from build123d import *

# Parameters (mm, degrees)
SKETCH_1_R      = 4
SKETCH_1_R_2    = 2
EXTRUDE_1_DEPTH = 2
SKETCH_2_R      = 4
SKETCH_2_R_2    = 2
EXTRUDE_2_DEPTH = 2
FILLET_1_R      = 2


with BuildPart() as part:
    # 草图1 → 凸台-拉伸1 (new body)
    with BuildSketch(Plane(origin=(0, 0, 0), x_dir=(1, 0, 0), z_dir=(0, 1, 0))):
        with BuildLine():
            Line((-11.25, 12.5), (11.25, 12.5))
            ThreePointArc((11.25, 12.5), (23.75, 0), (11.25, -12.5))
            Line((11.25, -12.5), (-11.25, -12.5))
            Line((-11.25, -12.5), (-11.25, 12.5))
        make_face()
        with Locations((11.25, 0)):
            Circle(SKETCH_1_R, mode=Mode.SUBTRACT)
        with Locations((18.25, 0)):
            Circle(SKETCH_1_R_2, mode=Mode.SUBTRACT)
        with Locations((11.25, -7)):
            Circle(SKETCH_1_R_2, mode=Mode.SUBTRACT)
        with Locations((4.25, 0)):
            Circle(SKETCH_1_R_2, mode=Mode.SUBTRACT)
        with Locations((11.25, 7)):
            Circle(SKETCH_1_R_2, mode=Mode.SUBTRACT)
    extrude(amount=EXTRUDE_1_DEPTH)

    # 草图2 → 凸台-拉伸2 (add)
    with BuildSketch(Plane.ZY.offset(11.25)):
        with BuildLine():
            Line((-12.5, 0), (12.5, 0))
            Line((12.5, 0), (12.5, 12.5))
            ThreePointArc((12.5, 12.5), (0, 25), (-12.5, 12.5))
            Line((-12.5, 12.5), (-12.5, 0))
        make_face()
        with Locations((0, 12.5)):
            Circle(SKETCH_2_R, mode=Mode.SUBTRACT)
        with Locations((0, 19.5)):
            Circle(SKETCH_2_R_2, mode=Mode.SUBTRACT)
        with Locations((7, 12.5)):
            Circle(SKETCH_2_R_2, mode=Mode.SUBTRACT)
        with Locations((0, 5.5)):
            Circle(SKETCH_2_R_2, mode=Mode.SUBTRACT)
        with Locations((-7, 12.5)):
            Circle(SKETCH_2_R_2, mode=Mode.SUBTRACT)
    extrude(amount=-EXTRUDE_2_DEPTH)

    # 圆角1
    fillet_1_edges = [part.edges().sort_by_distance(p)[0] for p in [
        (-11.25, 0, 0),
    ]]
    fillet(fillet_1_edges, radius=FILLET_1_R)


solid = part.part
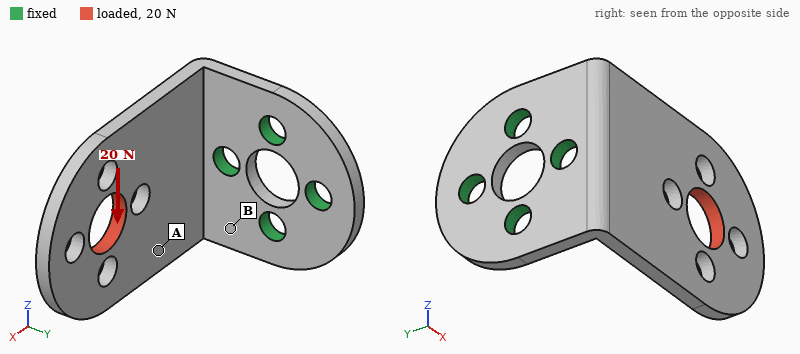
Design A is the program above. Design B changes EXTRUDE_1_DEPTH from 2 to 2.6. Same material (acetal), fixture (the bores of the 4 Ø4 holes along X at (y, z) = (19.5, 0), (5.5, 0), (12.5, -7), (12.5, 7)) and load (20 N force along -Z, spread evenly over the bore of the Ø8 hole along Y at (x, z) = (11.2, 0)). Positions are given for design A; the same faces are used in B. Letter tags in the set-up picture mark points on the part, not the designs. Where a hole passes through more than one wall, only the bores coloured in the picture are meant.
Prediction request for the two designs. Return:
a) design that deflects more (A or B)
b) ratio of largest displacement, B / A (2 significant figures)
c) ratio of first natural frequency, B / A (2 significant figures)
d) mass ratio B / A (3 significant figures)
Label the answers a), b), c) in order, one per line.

a) A
b) 0.77
c) 1.1
d) 1.18
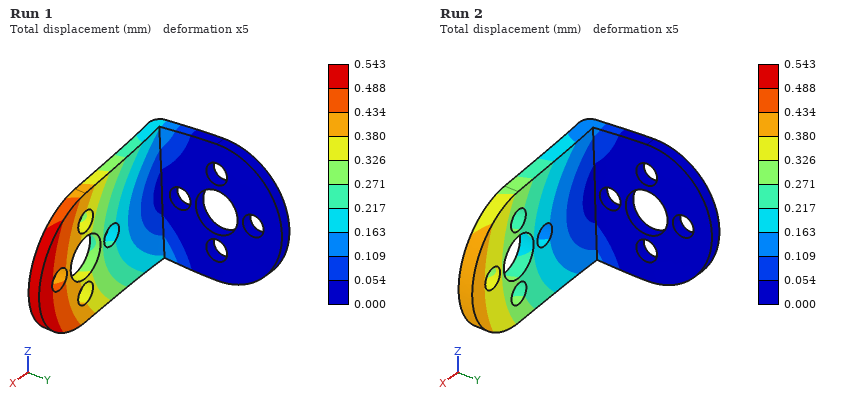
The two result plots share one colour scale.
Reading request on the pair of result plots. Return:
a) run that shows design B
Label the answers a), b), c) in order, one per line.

a) Run 2
